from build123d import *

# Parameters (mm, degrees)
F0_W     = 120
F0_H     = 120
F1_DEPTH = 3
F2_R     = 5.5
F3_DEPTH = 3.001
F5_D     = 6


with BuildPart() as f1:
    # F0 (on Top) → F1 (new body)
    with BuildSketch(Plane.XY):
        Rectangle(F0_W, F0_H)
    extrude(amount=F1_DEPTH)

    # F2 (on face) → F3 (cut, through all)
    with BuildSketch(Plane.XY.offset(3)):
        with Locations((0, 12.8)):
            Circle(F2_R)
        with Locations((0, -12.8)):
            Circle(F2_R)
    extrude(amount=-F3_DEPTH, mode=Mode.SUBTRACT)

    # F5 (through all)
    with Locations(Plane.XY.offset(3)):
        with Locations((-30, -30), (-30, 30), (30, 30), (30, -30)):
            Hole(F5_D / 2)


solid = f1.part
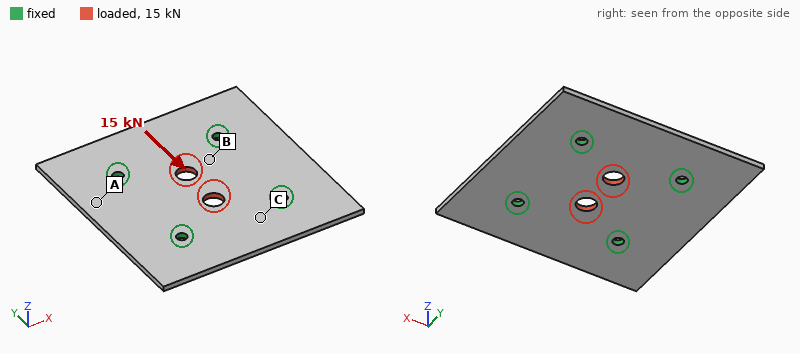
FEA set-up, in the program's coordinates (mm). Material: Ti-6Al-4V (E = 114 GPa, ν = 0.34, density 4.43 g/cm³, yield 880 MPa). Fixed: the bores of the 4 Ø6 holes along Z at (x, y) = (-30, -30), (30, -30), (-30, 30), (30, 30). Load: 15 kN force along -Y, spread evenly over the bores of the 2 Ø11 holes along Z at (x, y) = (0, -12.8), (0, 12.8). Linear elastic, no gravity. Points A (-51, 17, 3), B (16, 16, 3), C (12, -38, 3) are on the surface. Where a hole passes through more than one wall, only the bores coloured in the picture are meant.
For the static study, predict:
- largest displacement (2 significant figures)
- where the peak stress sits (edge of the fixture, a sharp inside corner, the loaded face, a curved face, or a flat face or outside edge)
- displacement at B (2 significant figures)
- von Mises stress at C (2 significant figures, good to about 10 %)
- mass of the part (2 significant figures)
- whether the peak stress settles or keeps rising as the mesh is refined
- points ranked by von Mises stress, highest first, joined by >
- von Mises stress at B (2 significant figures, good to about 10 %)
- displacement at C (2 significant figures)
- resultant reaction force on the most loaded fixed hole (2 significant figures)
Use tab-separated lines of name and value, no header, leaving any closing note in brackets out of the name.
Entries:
largest displacement	27 µm
where the peak stress sits	edge of the fixture
displacement at B	12 µm
von Mises stress at C	30 MPa
mass of the part	190 g
whether the peak stress settles or keeps rising as the mesh is refined	keeps rising
points ranked by von Mises stress, highest first, joined by >	B > C > A
von Mises stress at B	54 MPa
displacement at C	11 µm
resultant reaction force on the most loaded fixed hole	3.9 kN
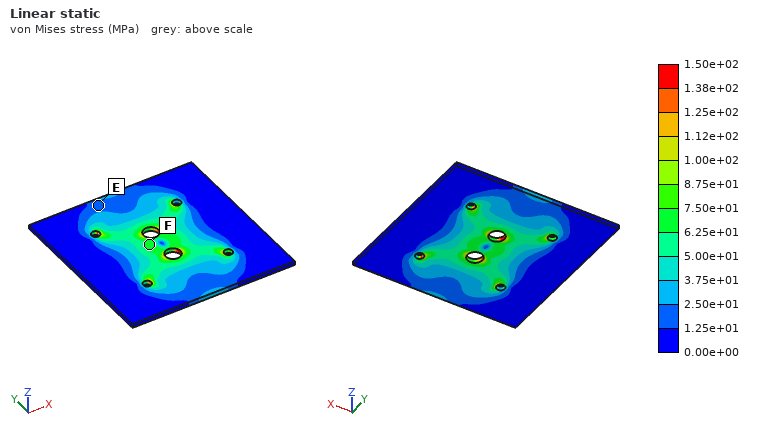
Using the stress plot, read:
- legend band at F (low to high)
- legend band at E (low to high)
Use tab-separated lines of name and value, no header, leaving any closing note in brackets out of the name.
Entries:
legend band at F	6.25e+01 to 7.50e+01 MPa
legend band at E	1.25e+01 to 2.50e+01 MPa
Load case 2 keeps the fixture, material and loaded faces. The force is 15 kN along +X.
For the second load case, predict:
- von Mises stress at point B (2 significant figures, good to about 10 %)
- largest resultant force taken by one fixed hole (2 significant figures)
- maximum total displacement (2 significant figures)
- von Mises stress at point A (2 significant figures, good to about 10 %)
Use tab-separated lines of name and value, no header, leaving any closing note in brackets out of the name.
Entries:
von Mises stress at point B	54 MPa
largest resultant force taken by one fixed hole	3.9 kN
maximum total displacement	21 µm
von Mises stress at point A	17 MPa
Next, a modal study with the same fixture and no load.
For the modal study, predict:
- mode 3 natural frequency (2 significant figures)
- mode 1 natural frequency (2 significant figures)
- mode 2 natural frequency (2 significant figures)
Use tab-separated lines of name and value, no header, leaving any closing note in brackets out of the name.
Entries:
mode 3 natural frequency	2300 Hz
mode 1 natural frequency	2200 Hz
mode 2 natural frequency	2300 Hz
